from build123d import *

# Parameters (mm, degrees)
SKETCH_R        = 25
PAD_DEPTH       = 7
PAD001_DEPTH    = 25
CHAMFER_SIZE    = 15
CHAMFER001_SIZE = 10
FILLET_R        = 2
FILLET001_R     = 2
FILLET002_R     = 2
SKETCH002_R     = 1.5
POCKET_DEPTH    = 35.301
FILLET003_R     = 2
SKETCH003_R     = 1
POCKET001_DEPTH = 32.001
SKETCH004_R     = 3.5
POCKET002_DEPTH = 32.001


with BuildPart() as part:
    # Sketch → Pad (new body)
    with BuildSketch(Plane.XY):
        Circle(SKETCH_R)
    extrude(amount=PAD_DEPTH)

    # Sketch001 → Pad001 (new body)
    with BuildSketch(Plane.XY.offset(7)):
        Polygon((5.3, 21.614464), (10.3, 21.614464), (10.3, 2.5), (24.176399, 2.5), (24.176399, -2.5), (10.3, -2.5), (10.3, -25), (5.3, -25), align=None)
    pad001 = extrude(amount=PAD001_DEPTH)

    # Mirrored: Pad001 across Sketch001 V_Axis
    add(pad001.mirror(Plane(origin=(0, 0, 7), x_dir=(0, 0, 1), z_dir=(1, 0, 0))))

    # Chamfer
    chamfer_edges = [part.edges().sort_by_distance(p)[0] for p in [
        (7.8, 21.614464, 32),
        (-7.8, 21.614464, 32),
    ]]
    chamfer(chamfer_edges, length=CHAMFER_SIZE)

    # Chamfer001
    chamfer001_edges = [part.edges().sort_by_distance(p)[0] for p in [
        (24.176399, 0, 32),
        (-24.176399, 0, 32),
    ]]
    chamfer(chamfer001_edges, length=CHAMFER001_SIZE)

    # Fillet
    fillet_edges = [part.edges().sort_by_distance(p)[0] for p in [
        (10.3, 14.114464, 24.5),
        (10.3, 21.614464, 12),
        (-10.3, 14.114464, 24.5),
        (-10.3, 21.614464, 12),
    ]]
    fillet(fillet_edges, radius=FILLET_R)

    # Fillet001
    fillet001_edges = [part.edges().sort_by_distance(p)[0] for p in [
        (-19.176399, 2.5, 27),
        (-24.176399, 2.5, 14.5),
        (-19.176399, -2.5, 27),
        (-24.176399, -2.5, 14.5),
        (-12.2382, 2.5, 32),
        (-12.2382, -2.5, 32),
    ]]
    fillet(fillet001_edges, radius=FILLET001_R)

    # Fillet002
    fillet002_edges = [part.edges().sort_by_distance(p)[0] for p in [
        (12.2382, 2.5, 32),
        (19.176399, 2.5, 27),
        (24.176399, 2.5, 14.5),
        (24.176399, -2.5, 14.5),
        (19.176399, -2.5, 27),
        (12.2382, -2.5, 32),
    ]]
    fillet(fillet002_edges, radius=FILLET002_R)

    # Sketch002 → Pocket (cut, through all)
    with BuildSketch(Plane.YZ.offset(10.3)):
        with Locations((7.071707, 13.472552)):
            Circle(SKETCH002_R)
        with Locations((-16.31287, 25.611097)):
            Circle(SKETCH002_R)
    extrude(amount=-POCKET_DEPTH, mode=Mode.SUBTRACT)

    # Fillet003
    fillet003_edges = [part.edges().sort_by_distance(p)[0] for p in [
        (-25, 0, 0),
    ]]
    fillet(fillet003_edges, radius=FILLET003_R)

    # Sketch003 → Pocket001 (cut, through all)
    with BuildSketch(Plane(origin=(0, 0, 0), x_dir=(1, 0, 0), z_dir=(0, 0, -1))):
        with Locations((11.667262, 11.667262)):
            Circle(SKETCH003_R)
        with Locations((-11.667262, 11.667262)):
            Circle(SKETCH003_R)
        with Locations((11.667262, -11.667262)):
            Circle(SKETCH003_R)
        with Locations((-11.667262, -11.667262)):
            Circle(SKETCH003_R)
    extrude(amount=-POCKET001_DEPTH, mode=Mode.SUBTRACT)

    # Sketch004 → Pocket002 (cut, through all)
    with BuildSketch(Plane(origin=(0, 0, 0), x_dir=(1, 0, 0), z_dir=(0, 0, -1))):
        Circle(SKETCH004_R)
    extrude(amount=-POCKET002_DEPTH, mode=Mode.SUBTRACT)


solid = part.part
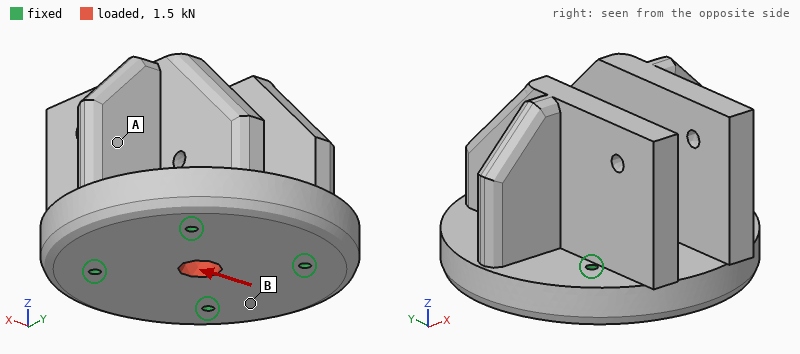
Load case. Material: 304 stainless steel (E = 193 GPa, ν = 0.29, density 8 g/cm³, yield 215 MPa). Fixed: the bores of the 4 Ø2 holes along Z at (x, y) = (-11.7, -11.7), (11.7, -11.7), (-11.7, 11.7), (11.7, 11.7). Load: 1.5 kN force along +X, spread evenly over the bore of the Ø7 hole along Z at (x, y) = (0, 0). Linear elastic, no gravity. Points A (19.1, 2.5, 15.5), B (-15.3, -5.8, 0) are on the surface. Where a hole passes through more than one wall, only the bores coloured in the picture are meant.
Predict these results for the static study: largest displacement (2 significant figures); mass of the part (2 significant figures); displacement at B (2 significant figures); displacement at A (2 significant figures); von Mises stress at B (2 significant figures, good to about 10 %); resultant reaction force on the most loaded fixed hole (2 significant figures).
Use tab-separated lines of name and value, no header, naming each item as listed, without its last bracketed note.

largest displacement	0.63 µm
mass of the part	210 g
displacement at B	0.23 µm
displacement at A	0.30 µm
von Mises stress at B	3.0 MPa
resultant reaction force on the most loaded fixed hole	390 N
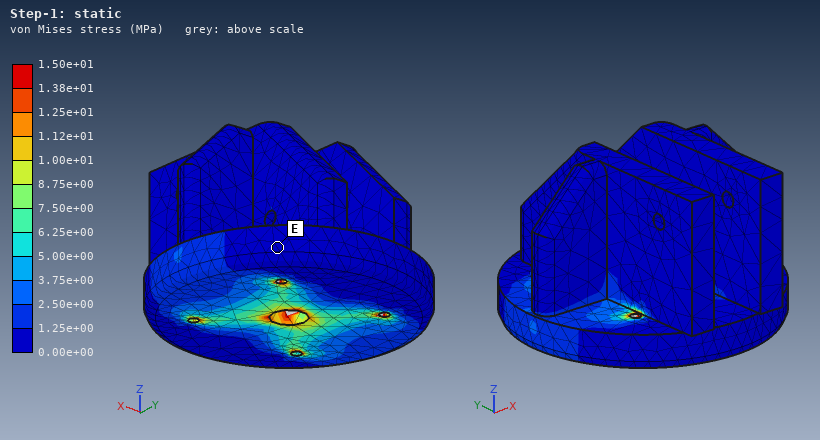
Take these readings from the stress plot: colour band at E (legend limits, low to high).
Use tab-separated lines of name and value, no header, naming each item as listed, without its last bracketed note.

colour band at E	0.00e+00 to 1.25e+00 MPa
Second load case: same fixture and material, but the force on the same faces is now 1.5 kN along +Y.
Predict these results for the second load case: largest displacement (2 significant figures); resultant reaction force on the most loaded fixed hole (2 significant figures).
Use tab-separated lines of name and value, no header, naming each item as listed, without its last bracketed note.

largest displacement	0.61 µm
resultant reaction force on the most loaded fixed hole	390 N
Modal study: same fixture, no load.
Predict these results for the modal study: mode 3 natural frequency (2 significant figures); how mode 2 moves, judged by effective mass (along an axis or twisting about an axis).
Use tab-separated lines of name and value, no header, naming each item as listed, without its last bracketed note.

mode 3 natural frequency	11 kHz
how mode 2 moves, judged by effective mass	along X
